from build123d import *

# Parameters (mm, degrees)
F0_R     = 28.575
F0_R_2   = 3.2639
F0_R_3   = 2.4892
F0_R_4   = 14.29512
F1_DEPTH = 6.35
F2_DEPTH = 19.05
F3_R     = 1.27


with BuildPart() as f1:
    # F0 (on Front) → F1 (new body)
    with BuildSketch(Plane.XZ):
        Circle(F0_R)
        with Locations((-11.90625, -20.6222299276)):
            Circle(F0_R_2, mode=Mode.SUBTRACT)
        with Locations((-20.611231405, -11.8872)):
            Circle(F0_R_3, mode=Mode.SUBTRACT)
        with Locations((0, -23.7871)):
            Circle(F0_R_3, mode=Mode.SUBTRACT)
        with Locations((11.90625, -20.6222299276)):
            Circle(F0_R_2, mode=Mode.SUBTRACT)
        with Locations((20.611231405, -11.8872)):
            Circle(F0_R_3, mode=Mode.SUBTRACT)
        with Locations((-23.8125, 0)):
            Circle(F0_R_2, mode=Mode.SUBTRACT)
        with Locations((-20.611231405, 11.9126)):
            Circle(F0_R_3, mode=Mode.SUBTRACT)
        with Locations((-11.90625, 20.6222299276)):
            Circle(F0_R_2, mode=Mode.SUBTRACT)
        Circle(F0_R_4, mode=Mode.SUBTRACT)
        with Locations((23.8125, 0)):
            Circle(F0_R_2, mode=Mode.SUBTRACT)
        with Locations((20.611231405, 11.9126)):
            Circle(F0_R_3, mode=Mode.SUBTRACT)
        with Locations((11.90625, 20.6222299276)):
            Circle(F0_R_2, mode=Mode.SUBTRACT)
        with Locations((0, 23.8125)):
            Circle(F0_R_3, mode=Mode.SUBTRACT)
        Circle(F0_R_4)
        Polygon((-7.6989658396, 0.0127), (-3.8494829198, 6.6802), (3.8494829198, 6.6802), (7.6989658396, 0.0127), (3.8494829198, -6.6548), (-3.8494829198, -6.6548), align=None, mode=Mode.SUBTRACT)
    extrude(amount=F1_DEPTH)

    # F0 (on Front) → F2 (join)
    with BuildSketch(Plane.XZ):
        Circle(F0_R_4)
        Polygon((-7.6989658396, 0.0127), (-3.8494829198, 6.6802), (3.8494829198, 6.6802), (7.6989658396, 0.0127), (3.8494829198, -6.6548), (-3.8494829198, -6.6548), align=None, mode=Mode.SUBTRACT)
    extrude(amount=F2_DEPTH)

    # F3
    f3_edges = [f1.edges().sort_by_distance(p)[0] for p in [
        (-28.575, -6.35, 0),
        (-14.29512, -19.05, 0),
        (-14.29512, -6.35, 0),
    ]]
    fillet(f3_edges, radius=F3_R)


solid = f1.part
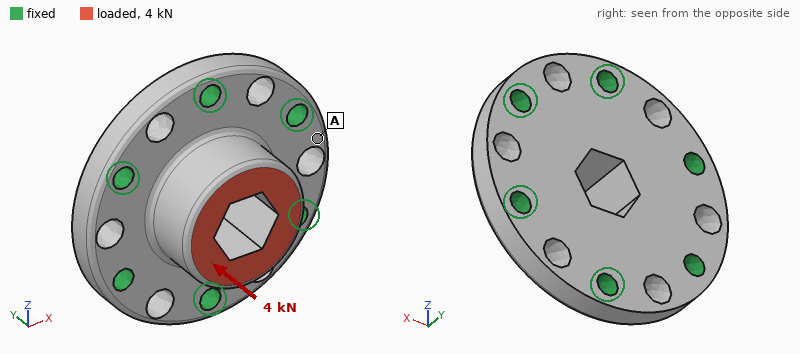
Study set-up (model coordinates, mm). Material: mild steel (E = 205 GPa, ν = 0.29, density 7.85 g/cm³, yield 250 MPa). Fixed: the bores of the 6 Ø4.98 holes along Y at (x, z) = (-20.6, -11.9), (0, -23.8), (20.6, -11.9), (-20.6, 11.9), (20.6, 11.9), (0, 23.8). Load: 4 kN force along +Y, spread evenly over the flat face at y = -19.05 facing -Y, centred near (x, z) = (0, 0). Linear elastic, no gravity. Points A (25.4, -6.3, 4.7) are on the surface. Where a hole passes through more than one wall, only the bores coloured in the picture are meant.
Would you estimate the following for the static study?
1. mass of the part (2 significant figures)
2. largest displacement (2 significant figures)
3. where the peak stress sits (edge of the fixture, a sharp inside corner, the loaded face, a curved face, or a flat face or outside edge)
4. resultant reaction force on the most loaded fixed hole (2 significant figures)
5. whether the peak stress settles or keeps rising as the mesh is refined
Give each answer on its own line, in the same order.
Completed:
150 g
3.0 µm
edge of the fixture
740 N
keeps rising
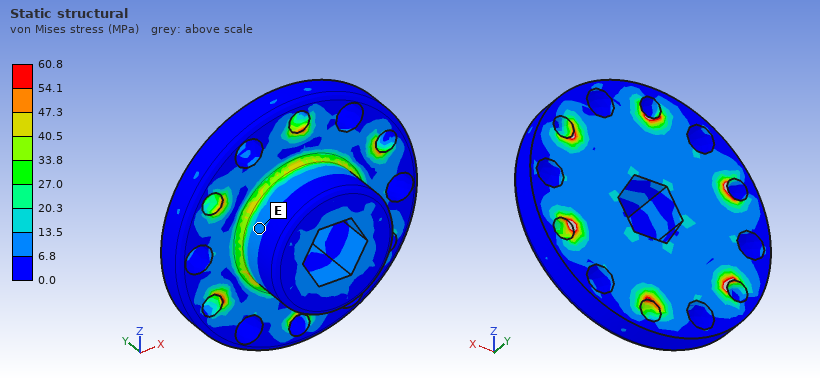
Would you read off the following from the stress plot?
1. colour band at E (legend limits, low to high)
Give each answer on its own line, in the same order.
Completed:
6.8 to 13.5 MPa
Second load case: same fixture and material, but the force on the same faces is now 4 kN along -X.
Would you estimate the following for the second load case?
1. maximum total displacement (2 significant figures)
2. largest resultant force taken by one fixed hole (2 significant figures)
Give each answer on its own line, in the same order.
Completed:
7.1 µm
1.3 kN
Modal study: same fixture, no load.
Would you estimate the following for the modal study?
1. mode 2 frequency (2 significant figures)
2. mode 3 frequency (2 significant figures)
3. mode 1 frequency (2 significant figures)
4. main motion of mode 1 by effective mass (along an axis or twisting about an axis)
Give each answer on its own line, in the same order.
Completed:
25 kHz
25 kHz
22 kHz
along Y
